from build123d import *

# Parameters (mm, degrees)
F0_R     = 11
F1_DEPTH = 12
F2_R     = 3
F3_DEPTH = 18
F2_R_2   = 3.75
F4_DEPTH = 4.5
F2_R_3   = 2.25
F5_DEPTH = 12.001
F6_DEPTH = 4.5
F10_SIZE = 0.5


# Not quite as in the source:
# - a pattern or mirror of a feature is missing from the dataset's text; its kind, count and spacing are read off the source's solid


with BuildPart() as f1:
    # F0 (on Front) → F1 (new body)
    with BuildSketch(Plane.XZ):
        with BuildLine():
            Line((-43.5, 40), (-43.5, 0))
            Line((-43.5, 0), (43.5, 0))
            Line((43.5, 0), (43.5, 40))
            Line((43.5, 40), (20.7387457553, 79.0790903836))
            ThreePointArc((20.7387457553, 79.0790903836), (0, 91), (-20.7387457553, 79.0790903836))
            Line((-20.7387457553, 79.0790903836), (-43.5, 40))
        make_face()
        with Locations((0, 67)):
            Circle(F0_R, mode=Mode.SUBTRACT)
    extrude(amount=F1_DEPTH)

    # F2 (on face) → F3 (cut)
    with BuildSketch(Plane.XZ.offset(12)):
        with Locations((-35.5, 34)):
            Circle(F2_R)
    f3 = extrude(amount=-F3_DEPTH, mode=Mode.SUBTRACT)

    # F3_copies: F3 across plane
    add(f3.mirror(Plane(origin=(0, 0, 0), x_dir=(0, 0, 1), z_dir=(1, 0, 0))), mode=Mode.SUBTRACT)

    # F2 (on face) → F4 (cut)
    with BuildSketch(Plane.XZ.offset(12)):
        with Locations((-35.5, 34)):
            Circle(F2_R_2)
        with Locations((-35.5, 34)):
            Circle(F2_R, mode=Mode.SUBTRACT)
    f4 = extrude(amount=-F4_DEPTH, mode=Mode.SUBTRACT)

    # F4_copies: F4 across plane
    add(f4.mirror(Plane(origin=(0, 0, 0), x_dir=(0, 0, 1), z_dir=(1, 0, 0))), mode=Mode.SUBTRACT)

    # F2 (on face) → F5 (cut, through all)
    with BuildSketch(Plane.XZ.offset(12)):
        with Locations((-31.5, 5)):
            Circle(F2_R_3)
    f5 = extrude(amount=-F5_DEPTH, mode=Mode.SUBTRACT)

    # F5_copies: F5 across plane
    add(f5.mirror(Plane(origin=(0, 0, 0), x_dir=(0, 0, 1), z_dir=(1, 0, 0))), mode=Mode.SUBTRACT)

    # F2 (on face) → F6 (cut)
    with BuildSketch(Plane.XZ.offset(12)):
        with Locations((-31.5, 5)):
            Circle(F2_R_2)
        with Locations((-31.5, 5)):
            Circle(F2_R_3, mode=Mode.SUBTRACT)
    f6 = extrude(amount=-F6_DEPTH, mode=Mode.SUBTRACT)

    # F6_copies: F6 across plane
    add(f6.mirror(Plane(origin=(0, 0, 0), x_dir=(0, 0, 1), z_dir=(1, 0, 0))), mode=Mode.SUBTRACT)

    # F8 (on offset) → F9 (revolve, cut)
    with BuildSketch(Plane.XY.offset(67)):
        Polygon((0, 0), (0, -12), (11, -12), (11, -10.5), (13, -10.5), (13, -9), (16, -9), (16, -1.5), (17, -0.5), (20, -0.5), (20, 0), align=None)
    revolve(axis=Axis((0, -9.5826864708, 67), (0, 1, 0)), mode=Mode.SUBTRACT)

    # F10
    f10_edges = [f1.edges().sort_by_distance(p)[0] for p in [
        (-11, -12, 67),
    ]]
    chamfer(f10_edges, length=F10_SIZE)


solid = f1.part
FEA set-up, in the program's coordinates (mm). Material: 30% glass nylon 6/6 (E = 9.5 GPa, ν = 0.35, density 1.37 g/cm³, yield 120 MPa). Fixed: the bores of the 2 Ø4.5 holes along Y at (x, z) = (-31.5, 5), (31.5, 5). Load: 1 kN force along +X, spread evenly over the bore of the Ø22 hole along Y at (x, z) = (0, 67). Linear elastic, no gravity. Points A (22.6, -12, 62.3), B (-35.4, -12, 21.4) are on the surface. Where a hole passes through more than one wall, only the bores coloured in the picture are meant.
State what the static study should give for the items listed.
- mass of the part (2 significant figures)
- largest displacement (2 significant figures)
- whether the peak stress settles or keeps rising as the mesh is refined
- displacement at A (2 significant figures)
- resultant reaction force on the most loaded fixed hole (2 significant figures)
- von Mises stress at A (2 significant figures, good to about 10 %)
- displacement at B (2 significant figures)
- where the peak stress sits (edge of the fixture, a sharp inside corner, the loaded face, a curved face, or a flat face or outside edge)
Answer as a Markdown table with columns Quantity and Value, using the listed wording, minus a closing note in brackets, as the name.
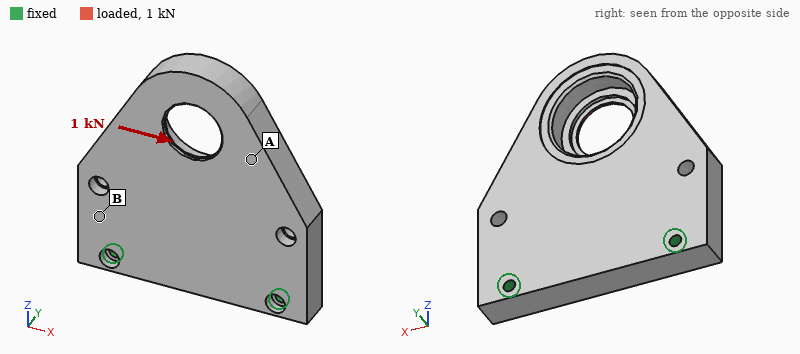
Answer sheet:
| Quantity | Value |
|---|---|
| mass of the part | 90 g |
| largest displacement | 0.10 mm |
| whether the peak stress settles or keeps rising as the mesh is refined | keeps rising |
| displacement at A | 0.062 mm |
| resultant reaction force on the most loaded fixed hole | 1.1 kN |
| von Mises stress at A | 6.1 MPa |
| displacement at B | 0.018 mm |
| where the peak stress sits | edge of the fixture |
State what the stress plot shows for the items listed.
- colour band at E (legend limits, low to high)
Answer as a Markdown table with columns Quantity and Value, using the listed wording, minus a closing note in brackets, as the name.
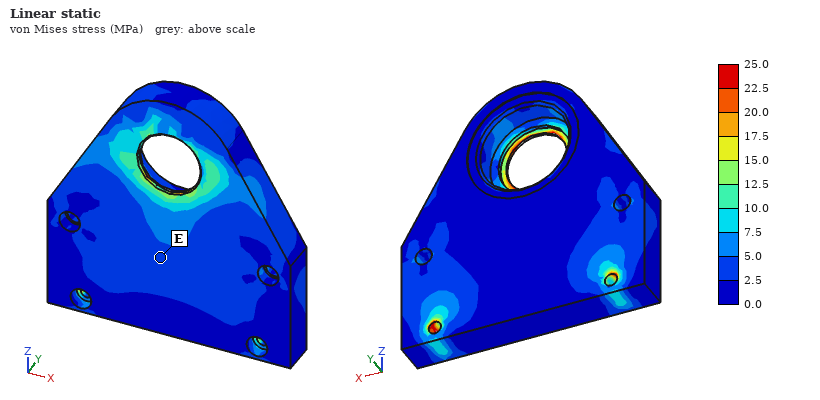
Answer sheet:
| Quantity | Value |
|---|---|
| colour band at E | 2.5 to 5.0 MPa |
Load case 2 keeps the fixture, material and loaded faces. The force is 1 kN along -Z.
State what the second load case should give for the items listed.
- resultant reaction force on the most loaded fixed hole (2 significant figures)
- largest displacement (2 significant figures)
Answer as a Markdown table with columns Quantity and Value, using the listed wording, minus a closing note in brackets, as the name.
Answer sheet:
| Quantity | Value |
|---|---|
| resultant reaction force on the most loaded fixed hole | 510 N |
| largest displacement | 0.38 mm |
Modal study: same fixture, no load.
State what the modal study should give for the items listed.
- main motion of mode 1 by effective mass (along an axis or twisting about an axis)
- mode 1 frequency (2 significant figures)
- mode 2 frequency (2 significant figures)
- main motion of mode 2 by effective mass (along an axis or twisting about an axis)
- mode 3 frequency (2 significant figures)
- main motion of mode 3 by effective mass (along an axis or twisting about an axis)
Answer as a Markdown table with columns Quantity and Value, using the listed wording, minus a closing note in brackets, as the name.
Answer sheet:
| Quantity | Value |
|---|---|
| main motion of mode 1 by effective mass | along Y |
| mode 1 frequency | 650 Hz |
| mode 2 frequency | 2200 Hz |
| main motion of mode 2 by effective mass | twisting about Z |
| mode 3 frequency | 3200 Hz |
| main motion of mode 3 by effective mass | along Y |
